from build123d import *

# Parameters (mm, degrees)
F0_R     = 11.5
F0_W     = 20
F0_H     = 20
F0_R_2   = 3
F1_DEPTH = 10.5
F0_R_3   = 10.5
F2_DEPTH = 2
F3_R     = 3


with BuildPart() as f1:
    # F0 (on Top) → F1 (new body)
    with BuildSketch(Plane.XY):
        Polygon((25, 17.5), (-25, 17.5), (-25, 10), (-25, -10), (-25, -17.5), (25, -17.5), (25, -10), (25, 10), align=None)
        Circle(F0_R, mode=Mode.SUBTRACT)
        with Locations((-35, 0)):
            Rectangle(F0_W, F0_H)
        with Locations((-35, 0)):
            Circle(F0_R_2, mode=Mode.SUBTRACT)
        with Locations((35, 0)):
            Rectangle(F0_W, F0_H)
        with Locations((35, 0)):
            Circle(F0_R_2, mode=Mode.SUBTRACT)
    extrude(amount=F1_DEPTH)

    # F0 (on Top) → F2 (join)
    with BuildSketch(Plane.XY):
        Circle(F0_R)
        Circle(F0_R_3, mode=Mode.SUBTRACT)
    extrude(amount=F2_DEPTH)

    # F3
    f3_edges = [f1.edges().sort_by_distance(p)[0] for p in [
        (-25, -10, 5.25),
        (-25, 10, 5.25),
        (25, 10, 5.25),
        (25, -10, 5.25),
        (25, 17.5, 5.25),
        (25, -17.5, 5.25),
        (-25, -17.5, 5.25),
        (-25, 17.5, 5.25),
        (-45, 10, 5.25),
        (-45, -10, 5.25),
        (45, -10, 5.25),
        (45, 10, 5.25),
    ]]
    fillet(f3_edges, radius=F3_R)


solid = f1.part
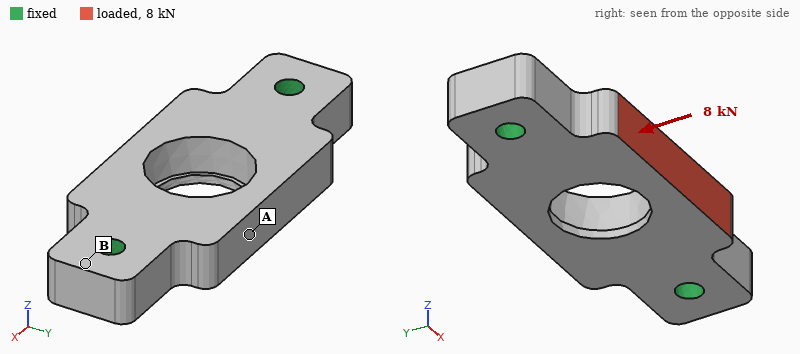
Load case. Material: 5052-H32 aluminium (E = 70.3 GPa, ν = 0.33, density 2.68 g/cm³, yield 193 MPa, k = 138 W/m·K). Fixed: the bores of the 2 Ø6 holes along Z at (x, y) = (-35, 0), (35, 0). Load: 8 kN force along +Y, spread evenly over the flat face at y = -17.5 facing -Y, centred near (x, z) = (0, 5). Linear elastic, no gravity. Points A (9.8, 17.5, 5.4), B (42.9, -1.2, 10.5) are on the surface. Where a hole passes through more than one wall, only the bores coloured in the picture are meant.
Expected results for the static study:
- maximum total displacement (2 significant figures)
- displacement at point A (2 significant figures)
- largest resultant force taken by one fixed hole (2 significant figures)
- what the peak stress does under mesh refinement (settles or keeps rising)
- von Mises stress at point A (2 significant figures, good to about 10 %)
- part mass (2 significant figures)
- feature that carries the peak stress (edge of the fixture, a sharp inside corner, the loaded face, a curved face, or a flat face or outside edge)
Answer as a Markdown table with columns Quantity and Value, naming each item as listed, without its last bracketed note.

| Quantity | Value |
|---|---|
| maximum total displacement | 39 µm |
| displacement at point A | 19 µm |
| largest resultant force taken by one fixed hole | 4.2 kN |
| what the peak stress does under mesh refinement | keeps rising |
| von Mises stress at point A | 32 MPa |
| part mass | 59 g |
| feature that carries the peak stress | edge of the fixture |
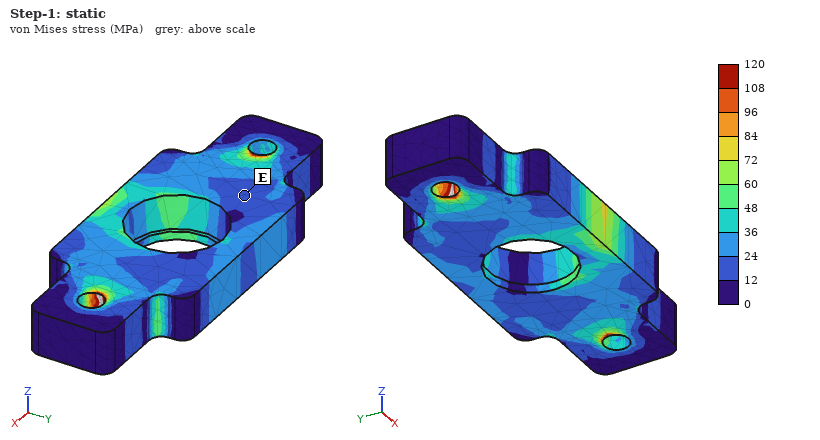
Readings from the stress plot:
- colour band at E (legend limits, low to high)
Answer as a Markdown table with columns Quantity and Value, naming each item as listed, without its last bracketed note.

| Quantity | Value |
|---|---|
| colour band at E | 12 to 24 MPa |
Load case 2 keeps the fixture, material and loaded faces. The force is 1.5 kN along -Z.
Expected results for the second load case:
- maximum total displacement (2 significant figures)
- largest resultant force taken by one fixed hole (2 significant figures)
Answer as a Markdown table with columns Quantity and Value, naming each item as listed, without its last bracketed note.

| Quantity | Value |
|---|---|
| maximum total displacement | 54 µm |
| largest resultant force taken by one fixed hole | 750 N |
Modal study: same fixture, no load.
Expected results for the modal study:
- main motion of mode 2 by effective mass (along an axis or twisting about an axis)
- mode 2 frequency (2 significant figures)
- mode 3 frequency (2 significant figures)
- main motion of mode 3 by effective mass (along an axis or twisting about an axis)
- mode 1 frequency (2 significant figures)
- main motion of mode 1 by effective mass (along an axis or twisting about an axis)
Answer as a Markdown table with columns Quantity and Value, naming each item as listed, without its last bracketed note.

| Quantity | Value |
|---|---|
| main motion of mode 2 by effective mass | twisting about X |
| mode 2 frequency | 9800 Hz |
| mode 3 frequency | 16 kHz |
| main motion of mode 3 by effective mass | along Y |
| mode 1 frequency | 9100 Hz |
| main motion of mode 1 by effective mass | along Z |
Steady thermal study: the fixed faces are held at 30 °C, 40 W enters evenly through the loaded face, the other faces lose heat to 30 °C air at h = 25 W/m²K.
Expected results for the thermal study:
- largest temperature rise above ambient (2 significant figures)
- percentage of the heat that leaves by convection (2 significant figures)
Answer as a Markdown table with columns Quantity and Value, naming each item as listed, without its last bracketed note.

| Quantity | Value |
|---|---|
| largest temperature rise above ambient | 25 K |
| percentage of the heat that leaves by convection | 3.3 % |
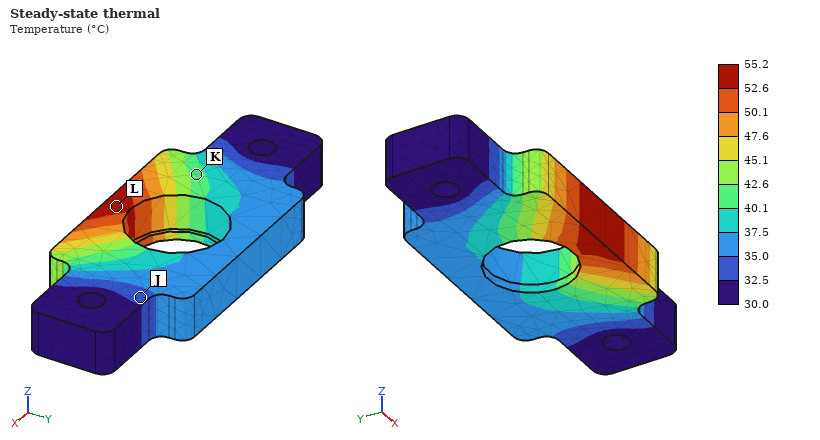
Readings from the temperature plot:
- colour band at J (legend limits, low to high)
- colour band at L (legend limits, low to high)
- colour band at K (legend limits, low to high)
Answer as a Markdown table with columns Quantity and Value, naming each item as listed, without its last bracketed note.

| Quantity | Value |
|---|---|
| colour band at J | 32.5 to 35.0 °C |
| colour band at L | 52.6 to 55.2 °C |
| colour band at K | 40.1 to 42.6 °C |
